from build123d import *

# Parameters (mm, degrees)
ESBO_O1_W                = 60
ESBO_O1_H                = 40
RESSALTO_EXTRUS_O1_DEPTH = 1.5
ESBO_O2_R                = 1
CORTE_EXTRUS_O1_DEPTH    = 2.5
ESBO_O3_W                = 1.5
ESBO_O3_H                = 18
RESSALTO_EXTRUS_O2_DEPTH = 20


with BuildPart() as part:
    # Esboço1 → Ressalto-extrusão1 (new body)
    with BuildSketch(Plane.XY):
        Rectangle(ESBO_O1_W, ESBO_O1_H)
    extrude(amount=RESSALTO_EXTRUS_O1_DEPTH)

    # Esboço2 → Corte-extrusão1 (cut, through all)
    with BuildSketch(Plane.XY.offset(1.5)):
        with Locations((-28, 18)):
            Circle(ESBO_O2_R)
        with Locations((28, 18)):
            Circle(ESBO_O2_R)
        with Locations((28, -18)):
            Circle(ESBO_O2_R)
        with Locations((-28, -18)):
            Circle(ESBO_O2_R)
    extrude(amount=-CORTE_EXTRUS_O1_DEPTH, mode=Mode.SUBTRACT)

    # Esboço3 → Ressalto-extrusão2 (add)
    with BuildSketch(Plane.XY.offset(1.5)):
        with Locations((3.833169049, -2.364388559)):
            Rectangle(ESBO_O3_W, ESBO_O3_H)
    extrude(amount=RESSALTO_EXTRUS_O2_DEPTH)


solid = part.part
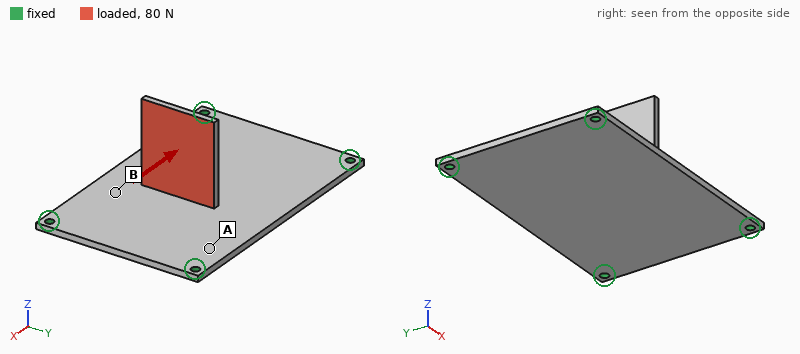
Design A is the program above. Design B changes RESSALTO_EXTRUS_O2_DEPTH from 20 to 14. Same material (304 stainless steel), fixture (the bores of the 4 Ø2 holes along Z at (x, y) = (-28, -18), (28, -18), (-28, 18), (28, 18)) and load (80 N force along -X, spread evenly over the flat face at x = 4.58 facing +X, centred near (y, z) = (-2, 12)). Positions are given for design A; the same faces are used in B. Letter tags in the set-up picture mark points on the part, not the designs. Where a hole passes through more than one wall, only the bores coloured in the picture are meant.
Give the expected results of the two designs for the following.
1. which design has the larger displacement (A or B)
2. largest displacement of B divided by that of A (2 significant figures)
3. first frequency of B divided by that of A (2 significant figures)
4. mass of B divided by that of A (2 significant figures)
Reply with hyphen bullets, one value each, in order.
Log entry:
- A
- 0.41
- 1.0
- 0.96
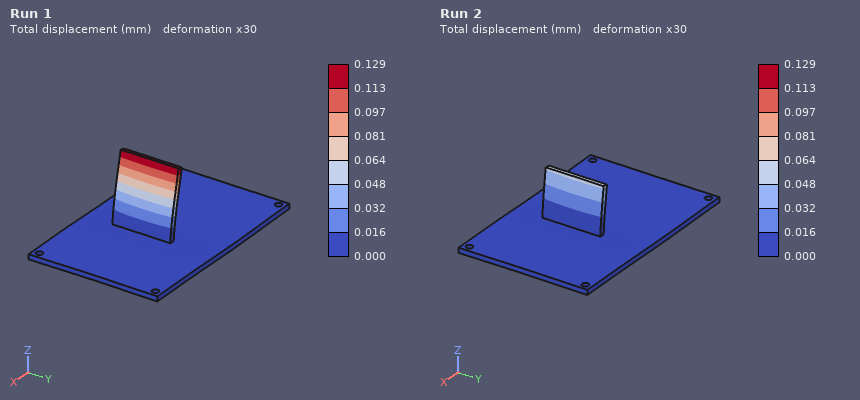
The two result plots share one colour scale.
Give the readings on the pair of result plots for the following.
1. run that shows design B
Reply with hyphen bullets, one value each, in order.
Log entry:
- Run 2
